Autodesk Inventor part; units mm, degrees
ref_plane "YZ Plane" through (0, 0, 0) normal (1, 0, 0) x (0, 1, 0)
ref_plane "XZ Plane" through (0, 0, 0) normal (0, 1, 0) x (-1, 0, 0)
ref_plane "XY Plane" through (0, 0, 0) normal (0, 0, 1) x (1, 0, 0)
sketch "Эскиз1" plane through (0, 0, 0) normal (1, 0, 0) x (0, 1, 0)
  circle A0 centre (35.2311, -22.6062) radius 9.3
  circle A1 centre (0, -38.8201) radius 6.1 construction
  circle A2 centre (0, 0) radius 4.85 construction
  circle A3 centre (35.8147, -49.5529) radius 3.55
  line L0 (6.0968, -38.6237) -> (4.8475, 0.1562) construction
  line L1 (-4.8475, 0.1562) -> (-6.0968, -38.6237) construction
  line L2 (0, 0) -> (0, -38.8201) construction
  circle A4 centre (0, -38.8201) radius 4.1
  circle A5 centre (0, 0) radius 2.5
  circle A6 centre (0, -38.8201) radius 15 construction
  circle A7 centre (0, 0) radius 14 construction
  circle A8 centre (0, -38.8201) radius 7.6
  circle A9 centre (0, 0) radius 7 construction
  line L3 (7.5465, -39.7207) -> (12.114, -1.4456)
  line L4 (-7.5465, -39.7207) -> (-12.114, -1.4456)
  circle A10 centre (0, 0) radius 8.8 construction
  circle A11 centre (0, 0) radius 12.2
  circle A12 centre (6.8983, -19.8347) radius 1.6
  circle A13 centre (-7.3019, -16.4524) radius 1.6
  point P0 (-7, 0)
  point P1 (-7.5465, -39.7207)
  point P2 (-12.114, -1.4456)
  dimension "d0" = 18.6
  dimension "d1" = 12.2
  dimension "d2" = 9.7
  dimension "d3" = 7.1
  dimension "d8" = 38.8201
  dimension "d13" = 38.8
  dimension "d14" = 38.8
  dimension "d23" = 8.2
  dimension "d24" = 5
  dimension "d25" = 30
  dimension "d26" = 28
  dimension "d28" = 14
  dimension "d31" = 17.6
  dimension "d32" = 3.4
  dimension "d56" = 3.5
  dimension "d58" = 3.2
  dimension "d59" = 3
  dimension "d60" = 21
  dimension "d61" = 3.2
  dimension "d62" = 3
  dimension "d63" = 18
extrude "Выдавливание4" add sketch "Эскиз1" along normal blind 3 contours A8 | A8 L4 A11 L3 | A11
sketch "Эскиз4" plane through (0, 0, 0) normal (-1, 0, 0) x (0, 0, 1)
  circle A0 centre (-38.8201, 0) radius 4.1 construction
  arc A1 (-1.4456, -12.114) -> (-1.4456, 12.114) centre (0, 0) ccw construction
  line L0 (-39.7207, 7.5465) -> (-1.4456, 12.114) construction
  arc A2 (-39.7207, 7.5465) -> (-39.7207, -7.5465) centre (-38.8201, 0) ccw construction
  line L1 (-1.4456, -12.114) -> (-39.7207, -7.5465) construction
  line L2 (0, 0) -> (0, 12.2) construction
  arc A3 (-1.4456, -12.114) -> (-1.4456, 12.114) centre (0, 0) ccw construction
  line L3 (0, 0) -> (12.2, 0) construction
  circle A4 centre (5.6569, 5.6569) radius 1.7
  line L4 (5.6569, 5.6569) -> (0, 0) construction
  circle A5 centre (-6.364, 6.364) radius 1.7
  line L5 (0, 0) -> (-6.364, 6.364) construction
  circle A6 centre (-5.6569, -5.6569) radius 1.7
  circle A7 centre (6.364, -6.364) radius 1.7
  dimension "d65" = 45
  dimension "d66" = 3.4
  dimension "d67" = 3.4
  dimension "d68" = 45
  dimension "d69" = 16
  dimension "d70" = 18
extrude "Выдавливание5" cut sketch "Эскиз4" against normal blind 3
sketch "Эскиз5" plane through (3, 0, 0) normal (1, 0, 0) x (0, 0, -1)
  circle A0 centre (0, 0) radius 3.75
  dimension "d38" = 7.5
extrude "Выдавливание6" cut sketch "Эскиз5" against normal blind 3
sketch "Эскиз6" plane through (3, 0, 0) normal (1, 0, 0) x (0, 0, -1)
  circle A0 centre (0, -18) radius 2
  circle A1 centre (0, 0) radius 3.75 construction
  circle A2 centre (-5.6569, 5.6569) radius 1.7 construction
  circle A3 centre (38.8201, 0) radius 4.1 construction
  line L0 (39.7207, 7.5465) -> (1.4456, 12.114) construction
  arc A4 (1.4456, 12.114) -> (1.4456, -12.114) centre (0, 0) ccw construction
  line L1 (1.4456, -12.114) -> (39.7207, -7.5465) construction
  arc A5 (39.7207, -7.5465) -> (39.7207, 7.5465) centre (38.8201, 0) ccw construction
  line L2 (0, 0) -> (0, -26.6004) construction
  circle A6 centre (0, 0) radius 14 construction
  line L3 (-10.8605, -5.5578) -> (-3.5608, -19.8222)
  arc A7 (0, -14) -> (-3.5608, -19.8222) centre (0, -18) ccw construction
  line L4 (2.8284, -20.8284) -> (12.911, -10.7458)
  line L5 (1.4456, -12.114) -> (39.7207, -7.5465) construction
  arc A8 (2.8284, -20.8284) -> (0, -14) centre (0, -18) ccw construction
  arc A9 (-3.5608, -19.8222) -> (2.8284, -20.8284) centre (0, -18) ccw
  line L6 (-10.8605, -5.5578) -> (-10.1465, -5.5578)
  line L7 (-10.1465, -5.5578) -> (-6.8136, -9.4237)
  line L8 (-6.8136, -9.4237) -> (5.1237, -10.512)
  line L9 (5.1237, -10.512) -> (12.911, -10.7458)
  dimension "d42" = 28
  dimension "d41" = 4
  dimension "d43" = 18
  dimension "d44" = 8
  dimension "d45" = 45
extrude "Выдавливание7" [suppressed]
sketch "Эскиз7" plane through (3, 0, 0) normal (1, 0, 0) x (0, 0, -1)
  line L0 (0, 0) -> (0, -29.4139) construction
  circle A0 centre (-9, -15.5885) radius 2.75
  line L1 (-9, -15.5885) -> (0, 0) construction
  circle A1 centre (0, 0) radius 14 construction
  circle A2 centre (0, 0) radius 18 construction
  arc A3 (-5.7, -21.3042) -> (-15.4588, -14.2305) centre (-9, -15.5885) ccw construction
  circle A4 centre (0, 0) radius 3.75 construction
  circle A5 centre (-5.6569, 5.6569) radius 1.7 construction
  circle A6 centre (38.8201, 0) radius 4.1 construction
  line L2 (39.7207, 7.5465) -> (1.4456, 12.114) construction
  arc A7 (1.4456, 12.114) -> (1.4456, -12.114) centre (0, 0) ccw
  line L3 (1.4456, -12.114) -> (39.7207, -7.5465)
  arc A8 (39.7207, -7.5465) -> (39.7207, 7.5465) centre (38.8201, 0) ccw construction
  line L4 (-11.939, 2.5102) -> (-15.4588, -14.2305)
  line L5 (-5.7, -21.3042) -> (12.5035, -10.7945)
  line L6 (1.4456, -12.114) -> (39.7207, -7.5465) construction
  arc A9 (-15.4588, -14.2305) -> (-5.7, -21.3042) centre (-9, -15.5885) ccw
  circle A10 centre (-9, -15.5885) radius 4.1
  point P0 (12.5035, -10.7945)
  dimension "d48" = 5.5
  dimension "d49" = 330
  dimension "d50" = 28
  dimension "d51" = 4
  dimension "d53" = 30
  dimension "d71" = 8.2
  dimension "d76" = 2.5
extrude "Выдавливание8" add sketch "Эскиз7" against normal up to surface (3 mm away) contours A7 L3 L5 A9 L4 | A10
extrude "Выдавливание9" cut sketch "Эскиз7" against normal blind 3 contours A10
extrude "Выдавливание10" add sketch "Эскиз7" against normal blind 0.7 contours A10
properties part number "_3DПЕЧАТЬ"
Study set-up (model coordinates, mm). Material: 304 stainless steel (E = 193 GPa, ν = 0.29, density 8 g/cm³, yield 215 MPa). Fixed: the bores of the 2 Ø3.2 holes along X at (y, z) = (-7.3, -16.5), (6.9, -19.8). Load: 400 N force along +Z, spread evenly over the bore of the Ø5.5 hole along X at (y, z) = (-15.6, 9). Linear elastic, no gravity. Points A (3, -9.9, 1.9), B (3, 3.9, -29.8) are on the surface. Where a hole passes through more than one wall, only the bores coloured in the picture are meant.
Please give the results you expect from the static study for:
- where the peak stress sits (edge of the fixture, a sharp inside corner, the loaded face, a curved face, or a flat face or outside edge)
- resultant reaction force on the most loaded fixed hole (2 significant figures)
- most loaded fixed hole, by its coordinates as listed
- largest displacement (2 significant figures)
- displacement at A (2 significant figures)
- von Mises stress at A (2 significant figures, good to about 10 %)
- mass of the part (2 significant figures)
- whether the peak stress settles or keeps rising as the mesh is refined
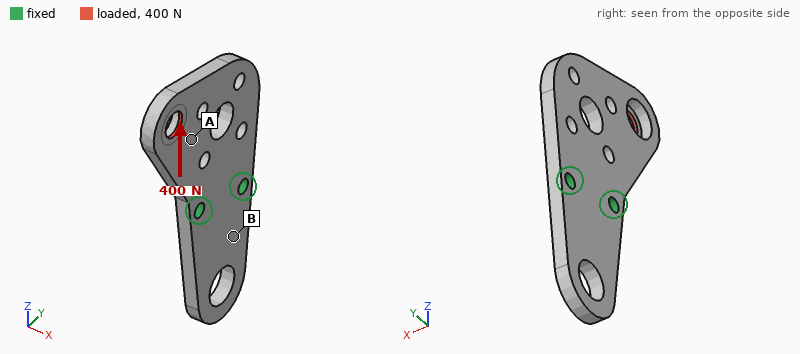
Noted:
a sharp inside corner
610 N
(-7.3, -16.5)
34 µm
12 µm
28 MPa
27 g
keeps rising
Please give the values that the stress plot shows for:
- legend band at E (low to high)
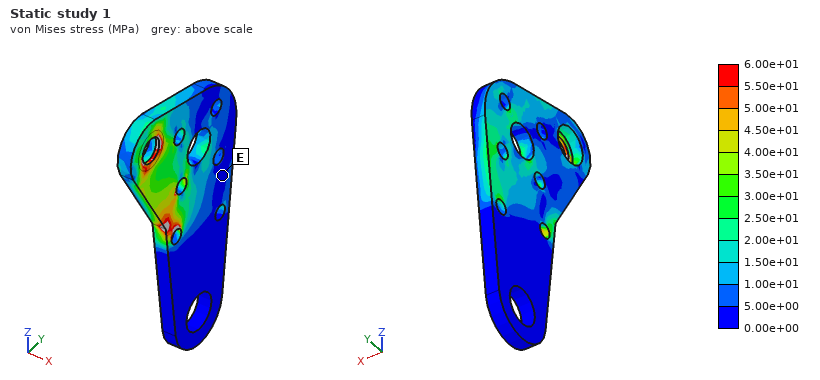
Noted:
0.00e+00 to 5.00e+00 MPa
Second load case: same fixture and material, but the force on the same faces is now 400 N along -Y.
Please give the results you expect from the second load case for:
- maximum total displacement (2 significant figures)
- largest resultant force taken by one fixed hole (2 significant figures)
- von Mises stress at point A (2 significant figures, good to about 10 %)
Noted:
25 µm
730 N
29 MPa
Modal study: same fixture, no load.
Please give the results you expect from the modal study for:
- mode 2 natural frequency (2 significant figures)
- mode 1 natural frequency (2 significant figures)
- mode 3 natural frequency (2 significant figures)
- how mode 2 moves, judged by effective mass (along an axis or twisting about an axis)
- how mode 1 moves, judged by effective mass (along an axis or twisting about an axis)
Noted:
4300 Hz
2300 Hz
5000 Hz
along X
along X
